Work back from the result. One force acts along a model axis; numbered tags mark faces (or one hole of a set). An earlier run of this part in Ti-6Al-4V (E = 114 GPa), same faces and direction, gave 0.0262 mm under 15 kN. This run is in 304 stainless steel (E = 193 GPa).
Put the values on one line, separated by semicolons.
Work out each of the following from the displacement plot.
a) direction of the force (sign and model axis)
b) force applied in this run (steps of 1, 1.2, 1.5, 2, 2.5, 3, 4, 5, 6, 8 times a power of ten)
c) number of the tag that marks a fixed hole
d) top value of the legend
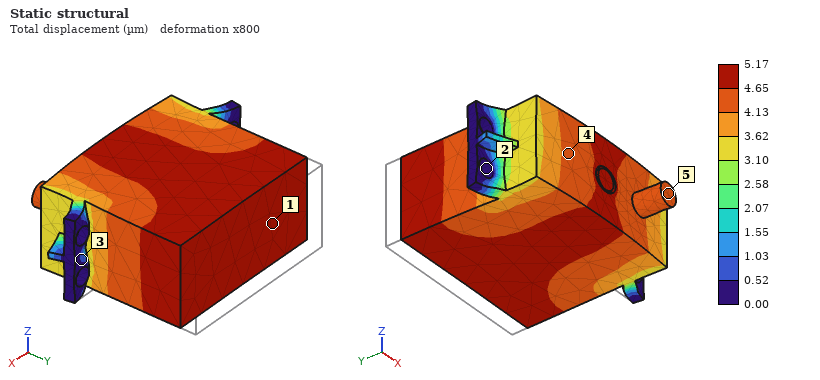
-Y; 5 kN; 2; 5.17 µm
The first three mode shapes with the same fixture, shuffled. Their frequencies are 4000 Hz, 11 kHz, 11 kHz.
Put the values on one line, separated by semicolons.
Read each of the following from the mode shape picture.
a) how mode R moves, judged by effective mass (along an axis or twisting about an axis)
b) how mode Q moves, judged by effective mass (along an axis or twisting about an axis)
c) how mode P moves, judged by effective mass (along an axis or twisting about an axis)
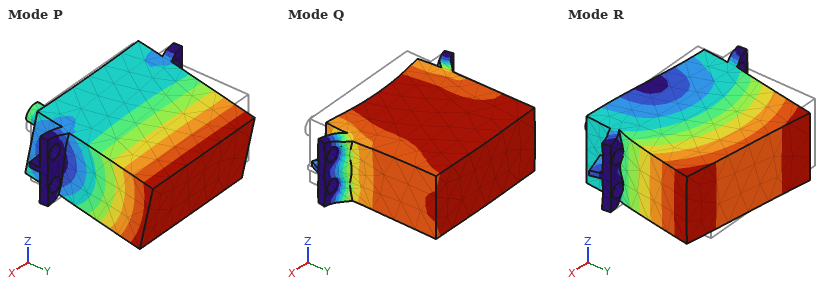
along X; along Y; along Z
